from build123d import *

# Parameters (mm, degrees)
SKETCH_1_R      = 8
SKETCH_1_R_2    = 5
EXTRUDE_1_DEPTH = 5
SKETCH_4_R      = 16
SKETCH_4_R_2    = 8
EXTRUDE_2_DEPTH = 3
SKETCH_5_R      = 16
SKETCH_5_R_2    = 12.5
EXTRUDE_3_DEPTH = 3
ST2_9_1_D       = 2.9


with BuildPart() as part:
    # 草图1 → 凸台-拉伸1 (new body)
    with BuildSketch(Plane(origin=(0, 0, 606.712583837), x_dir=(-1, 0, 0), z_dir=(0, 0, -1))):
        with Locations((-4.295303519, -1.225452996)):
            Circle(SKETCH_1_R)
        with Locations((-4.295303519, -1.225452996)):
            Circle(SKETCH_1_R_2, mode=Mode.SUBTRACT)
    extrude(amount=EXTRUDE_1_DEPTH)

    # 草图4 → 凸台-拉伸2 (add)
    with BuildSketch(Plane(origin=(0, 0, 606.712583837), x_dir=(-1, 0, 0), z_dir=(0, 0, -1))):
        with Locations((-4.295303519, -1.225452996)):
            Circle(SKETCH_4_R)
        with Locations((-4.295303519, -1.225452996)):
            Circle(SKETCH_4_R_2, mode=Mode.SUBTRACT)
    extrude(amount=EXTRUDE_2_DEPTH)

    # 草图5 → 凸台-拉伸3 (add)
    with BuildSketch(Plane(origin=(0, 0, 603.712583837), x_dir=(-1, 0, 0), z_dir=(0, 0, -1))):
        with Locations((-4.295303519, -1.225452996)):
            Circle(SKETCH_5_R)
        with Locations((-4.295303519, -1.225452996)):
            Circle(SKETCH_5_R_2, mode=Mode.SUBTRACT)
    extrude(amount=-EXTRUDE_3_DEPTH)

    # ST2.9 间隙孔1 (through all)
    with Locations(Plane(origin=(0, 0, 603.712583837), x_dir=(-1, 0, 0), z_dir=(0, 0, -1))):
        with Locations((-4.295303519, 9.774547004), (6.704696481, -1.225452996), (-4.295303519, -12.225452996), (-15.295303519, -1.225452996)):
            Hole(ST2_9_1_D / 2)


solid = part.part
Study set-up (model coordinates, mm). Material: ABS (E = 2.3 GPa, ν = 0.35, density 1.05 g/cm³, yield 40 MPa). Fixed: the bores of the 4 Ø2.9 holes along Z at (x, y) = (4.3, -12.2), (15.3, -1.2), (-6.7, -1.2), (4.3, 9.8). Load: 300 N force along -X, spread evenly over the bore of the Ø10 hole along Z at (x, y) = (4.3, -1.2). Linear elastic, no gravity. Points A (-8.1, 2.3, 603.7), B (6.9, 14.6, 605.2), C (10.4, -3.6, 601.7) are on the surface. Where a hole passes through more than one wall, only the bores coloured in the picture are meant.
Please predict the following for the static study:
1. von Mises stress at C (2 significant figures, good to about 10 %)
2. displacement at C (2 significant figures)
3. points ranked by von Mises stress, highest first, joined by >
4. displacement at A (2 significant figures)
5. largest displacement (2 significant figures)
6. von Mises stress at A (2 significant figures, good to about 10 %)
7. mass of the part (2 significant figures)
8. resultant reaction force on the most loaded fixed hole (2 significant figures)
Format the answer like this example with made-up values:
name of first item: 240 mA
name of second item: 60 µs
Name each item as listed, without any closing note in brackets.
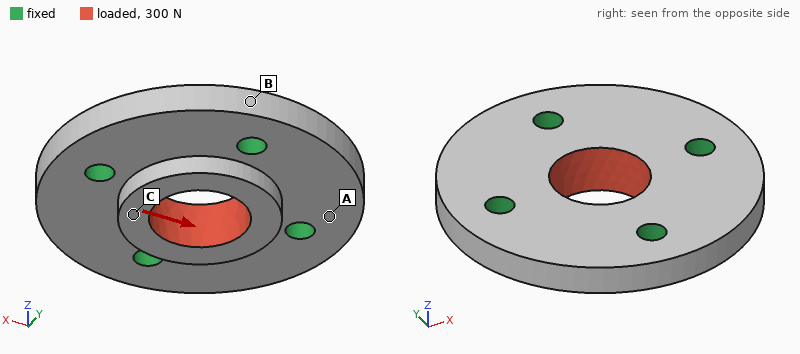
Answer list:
von Mises stress at C: 2.6 MPa
displacement at C: 14 µm
points ranked by von Mises stress, highest first, joined by >: C > A > B
displacement at A: 3.3 µm
largest displacement: 16 µm
von Mises stress at A: 1.7 MPa
mass of the part: 2.5 g
resultant reaction force on the most loaded fixed hole: 90 N
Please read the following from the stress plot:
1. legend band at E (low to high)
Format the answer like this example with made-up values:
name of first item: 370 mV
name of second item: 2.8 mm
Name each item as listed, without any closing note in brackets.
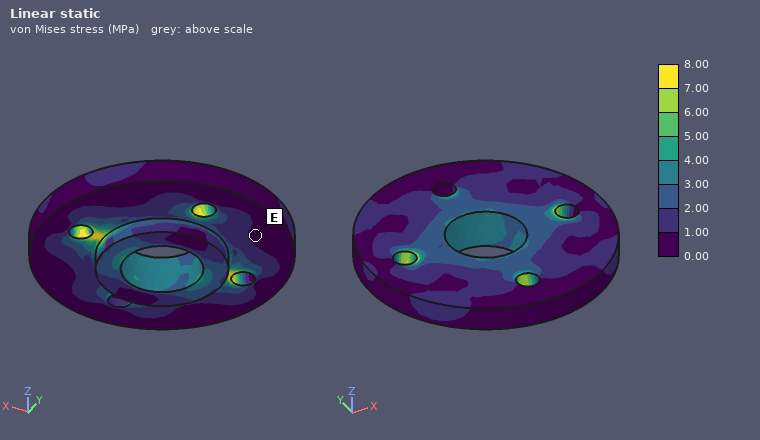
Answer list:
legend band at E: 0.00 to 1.00 MPa
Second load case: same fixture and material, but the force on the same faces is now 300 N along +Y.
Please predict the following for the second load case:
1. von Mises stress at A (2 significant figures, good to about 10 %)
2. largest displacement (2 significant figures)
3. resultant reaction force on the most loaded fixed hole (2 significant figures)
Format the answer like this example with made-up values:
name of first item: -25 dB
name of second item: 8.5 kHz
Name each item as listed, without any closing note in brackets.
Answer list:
von Mises stress at A: 1.3 MPa
largest displacement: 16 µm
resultant reaction force on the most loaded fixed hole: 90 N
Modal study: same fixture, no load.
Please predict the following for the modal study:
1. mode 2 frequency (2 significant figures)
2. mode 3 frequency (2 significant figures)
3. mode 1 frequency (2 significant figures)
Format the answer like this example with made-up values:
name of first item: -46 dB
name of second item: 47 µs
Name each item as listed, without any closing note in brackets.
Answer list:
mode 2 frequency: 11 kHz
mode 3 frequency: 11 kHz
mode 1 frequency: 10 kHz
